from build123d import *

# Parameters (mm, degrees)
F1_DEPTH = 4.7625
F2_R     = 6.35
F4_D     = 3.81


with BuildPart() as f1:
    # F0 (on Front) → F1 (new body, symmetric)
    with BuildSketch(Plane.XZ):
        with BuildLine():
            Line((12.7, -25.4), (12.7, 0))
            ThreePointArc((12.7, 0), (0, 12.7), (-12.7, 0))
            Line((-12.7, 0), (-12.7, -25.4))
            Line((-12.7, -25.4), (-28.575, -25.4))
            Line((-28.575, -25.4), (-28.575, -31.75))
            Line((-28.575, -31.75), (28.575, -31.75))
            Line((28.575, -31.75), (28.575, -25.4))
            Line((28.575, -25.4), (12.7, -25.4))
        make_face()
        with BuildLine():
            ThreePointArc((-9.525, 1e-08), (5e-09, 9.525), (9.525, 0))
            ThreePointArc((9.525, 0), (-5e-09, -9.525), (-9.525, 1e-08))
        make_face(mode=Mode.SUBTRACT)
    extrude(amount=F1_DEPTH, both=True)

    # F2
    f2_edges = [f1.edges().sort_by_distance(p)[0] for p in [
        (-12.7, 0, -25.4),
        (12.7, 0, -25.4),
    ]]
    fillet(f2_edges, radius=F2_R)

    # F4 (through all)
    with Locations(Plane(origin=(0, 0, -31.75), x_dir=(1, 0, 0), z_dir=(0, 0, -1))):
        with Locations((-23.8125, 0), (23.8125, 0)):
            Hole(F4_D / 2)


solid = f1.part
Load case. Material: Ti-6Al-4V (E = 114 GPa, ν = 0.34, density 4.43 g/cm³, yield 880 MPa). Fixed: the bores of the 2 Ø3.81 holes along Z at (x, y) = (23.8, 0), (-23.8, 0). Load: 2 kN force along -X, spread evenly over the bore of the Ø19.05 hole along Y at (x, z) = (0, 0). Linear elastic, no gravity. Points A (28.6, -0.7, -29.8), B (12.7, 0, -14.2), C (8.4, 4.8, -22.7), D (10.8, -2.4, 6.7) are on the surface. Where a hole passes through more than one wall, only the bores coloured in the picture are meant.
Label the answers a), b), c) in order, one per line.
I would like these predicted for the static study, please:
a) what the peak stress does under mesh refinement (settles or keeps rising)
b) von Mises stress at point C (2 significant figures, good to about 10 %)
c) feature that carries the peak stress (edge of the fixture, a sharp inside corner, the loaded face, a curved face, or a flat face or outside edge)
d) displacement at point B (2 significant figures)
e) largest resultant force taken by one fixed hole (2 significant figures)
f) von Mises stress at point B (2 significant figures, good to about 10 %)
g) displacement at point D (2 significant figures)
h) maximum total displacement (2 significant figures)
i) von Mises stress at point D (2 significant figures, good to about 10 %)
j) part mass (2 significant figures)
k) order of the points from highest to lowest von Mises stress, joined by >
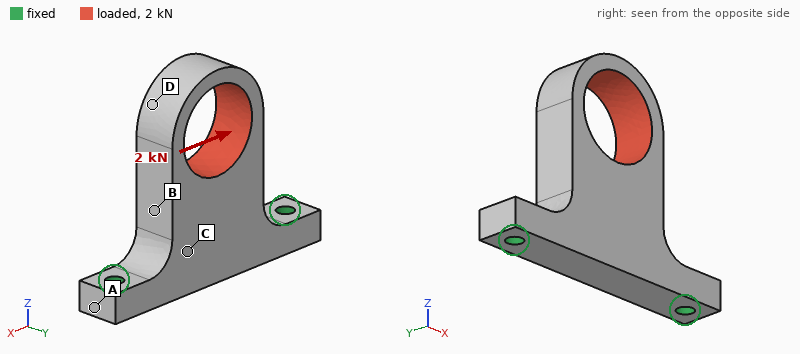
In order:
a) keeps rising
b) 21 MPa
c) edge of the fixture
d) 19 µm
e) 1.8 kN
f) 52 MPa
g) 87 µm
h) 95 µm
i) 70 MPa
j) 41 g
k) D > B > C > A
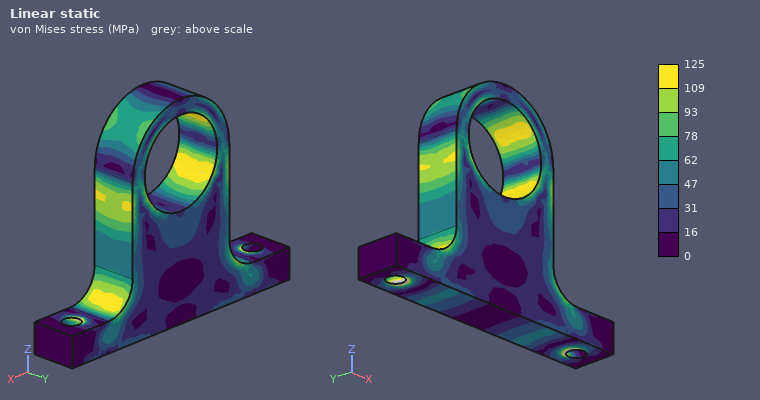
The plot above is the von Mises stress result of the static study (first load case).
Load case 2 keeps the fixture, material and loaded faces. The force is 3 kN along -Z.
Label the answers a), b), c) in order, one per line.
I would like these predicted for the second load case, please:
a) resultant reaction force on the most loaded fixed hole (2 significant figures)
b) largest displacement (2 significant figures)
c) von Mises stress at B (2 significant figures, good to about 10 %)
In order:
a) 1.7 kN
b) 33 µm
c) 35 MPa
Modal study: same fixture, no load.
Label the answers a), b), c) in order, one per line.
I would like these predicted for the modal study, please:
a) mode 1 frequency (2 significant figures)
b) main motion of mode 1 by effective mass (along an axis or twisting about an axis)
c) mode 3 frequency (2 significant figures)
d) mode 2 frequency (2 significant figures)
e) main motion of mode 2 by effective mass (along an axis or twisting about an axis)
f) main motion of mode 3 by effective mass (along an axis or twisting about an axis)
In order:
a) 2900 Hz
b) along Y
c) 12 kHz
d) 8200 Hz
e) along X
f) along Z
